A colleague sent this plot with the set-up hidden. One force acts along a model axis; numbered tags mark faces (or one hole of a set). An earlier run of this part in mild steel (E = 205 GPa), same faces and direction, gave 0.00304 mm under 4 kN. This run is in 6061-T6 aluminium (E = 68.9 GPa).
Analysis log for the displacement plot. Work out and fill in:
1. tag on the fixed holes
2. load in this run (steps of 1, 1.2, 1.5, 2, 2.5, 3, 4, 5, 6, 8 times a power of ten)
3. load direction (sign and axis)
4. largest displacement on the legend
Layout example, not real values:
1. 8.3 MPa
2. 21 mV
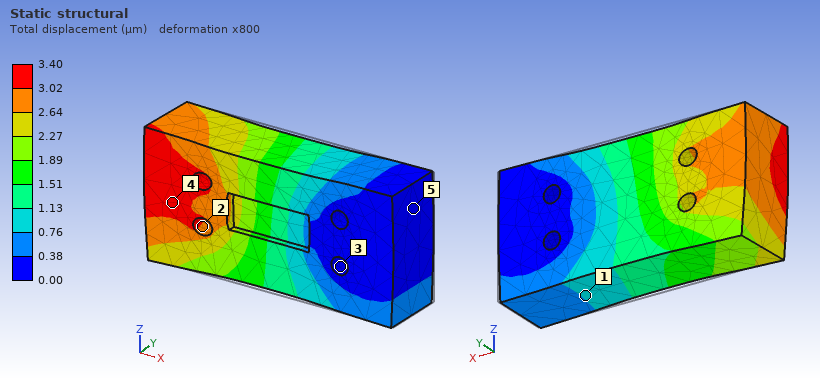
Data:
1. 3
2. 1.5 kN
3. -X
4. 3.40 µm
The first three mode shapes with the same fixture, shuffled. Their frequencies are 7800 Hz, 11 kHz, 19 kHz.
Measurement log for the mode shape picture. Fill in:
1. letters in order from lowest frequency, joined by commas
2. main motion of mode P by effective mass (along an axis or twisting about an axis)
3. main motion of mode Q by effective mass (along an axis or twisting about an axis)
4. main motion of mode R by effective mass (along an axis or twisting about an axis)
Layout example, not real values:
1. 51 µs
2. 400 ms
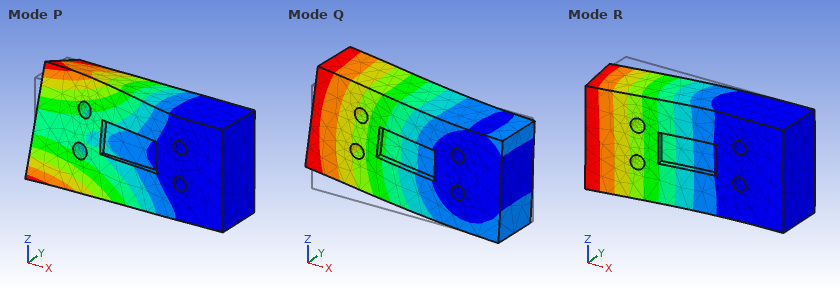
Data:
1. R, Q, P
2. twisting about X
3. along Z
4. along Y
